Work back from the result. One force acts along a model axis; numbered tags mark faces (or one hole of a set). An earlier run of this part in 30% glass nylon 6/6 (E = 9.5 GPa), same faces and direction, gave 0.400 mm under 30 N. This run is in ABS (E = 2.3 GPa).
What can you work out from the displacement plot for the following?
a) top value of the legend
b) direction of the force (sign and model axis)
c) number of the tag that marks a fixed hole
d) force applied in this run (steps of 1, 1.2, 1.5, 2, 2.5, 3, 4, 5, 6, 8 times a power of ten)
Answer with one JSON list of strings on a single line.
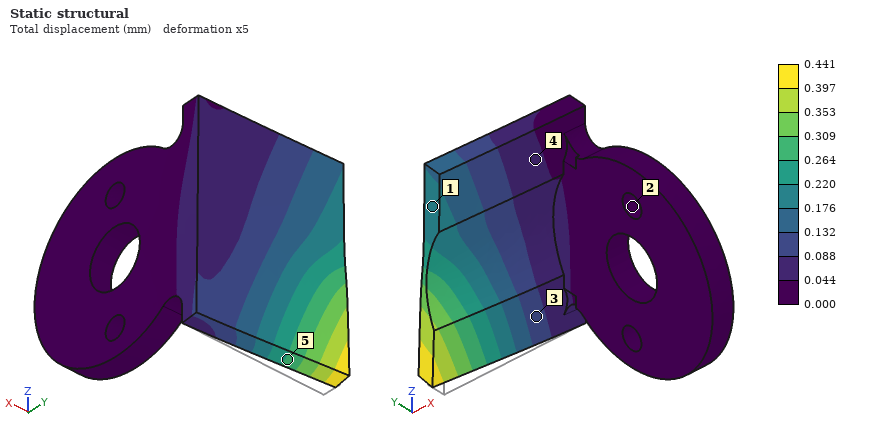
["0.441 mm", "+Y", "2", "8 N"]
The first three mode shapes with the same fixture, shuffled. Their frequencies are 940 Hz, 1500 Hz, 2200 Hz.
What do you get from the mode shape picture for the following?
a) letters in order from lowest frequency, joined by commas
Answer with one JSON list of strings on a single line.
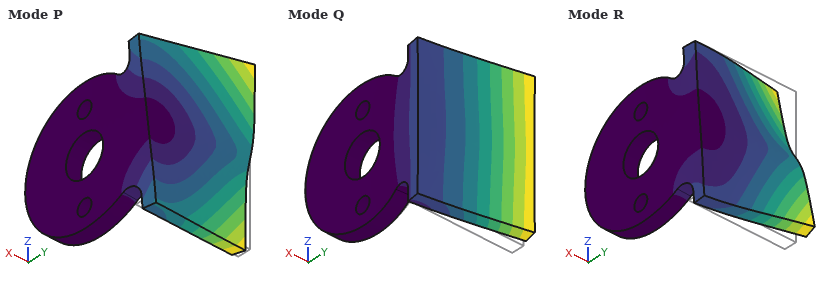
["Q, P, R"]
